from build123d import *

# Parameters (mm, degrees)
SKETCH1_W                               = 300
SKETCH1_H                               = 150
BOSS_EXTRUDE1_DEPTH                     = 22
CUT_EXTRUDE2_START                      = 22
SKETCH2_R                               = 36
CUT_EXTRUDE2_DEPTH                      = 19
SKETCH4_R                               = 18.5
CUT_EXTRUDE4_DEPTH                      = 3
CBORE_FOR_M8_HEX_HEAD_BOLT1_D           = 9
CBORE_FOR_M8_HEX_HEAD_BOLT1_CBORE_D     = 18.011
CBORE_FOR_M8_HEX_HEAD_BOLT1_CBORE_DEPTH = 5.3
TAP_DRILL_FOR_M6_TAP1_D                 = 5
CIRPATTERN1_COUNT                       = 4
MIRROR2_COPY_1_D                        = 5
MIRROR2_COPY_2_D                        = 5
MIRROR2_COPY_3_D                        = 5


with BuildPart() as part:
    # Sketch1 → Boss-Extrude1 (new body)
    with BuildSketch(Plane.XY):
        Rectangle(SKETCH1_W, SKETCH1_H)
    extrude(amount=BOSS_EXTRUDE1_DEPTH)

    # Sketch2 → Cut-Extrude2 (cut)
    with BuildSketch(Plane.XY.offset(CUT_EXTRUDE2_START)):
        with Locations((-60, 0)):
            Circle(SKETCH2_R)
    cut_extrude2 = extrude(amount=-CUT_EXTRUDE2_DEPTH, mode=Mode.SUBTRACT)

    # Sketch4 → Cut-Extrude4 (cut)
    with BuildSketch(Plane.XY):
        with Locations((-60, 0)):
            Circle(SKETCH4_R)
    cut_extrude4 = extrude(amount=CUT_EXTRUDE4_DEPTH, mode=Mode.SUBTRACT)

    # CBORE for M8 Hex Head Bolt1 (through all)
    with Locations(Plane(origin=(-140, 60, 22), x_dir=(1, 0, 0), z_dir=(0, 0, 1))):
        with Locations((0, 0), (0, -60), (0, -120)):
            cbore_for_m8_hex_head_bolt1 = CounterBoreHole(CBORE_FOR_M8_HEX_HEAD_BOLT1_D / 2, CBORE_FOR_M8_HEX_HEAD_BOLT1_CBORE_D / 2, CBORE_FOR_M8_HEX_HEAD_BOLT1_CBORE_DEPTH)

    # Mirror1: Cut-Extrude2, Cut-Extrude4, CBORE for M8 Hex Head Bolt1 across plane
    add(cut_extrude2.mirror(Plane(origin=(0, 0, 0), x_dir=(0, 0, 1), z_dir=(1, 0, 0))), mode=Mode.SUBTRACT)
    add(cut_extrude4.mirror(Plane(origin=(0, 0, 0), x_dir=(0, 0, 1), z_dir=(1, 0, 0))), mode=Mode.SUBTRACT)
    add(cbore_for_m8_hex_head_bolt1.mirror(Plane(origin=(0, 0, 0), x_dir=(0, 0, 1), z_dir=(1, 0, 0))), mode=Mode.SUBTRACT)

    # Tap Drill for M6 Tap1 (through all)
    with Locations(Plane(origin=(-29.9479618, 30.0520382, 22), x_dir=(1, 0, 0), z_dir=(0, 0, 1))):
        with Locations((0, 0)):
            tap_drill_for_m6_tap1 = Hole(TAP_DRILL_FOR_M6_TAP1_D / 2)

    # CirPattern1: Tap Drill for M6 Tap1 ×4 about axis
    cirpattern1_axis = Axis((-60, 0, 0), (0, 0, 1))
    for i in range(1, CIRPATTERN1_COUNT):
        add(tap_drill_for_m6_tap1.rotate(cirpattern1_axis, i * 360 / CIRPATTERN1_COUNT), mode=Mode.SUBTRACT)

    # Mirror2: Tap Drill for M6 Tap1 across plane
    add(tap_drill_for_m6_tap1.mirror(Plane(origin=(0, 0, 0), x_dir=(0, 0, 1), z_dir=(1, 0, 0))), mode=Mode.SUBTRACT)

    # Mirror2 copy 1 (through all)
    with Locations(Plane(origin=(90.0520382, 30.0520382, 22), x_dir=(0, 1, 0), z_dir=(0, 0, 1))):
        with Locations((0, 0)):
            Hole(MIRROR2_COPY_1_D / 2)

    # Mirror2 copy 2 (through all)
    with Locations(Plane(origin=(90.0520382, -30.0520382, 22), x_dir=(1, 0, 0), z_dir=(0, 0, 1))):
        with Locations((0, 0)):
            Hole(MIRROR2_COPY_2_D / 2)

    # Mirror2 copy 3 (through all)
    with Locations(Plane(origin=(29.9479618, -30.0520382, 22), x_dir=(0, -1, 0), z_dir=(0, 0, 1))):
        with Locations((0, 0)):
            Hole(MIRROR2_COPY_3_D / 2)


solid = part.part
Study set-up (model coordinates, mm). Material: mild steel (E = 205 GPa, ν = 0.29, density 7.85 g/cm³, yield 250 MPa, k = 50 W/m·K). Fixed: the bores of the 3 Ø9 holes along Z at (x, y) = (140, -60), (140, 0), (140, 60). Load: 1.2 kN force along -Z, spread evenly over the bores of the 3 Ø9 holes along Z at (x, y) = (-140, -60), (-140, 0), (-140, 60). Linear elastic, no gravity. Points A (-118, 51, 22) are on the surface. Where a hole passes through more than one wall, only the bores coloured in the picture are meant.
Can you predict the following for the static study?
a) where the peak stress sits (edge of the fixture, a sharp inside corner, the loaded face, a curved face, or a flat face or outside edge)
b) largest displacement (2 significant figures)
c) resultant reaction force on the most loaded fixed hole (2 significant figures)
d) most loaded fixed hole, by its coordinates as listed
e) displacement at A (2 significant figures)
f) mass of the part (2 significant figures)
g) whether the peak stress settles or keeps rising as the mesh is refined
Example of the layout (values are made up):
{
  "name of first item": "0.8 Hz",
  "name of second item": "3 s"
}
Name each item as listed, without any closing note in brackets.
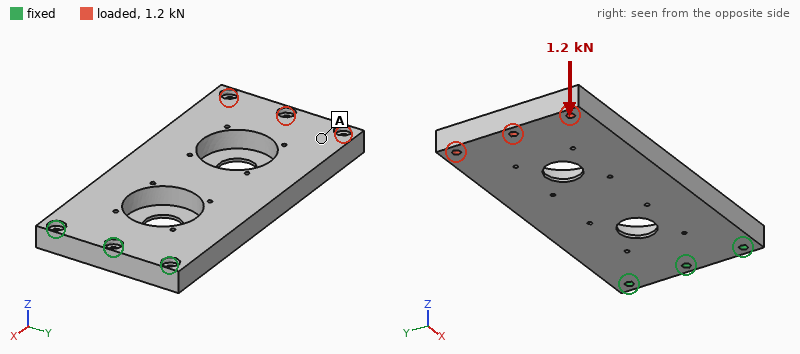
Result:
{
  "where the peak stress sits": "edge of the fixture",
  "largest displacement": "0.52 mm",
  "resultant reaction force on the most loaded fixed hole": "1.4 kN",
  "most loaded fixed hole, by its coordinates as listed": "(140, 0)",
  "displacement at A": "0.44 mm",
  "mass of the part": "6.4 kg",
  "whether the peak stress settles or keeps rising as the mesh is refined": "keeps rising"
}
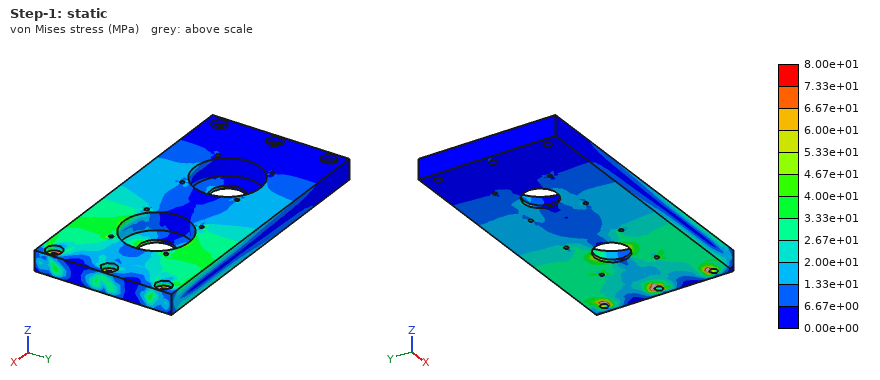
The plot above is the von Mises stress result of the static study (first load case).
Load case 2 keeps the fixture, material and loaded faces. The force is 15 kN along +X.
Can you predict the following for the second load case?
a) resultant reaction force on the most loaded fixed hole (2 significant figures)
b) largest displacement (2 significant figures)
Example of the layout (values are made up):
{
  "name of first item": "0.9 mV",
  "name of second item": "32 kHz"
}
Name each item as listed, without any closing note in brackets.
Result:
{
  "resultant reaction force on the most loaded fixed hole": "5.7 kN",
  "largest displacement": "66 µm"
}
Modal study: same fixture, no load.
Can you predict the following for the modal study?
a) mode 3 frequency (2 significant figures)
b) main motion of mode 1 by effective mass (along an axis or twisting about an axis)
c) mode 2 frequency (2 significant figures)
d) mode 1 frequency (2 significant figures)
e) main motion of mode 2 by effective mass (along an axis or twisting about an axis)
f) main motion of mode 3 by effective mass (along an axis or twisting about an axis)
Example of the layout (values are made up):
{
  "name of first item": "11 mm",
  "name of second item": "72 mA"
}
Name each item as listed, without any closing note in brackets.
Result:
{
  "mode 3 frequency": "1100 Hz",
  "main motion of mode 1 by effective mass": "along Z",
  "mode 2 frequency": "740 Hz",
  "mode 1 frequency": "190 Hz",
  "main motion of mode 2 by effective mass": "twisting about X",
  "main motion of mode 3 by effective mass": "along Y"
}
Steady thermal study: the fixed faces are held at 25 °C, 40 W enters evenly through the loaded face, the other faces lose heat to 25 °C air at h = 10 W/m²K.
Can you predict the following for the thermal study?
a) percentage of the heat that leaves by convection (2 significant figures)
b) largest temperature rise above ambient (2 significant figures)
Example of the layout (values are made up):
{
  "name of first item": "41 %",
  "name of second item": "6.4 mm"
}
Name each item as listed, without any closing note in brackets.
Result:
{
  "percentage of the heat that leaves by convection": "65 %",
  "largest temperature rise above ambient": "55 K"
}
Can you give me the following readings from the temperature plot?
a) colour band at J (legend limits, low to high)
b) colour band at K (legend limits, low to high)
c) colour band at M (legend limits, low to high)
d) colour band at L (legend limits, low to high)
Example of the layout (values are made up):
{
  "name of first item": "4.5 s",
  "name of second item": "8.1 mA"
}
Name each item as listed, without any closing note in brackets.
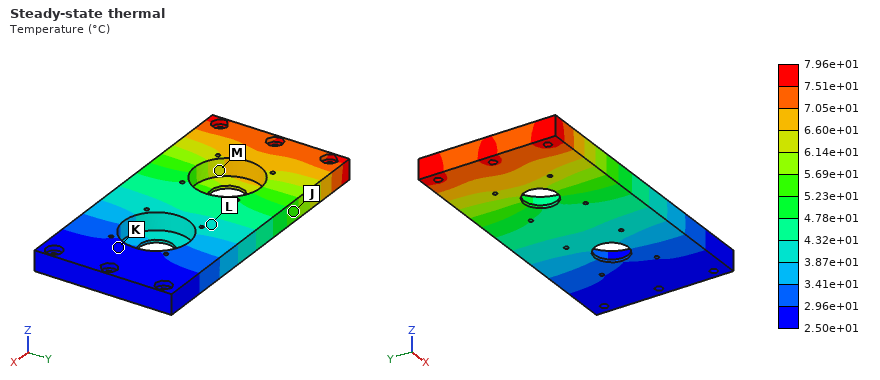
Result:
{
  "colour band at J": "5.23e+01 to 5.69e+01 °C",
  "colour band at K": "2.50e+01 to 2.96e+01 °C",
  "colour band at M": "6.14e+01 to 6.60e+01 °C",
  "colour band at L": "3.87e+01 to 4.32e+01 °C"
}
